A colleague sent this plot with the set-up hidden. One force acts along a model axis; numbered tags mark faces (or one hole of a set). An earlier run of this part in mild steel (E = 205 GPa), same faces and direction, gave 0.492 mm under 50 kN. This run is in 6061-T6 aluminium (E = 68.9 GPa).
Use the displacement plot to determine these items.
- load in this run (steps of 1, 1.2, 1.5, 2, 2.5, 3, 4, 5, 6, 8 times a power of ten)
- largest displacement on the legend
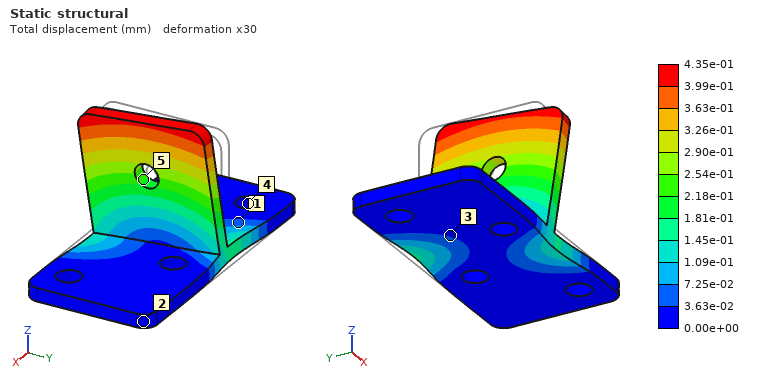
15 kN
4.35e-01 mm
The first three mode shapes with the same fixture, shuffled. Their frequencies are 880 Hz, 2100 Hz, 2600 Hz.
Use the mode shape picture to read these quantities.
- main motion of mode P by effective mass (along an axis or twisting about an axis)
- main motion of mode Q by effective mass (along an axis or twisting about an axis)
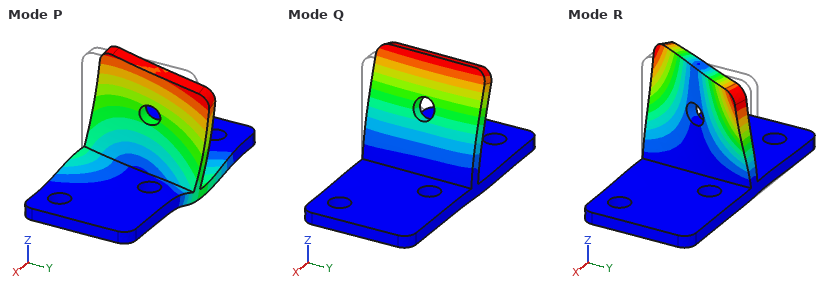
along Y
along X
